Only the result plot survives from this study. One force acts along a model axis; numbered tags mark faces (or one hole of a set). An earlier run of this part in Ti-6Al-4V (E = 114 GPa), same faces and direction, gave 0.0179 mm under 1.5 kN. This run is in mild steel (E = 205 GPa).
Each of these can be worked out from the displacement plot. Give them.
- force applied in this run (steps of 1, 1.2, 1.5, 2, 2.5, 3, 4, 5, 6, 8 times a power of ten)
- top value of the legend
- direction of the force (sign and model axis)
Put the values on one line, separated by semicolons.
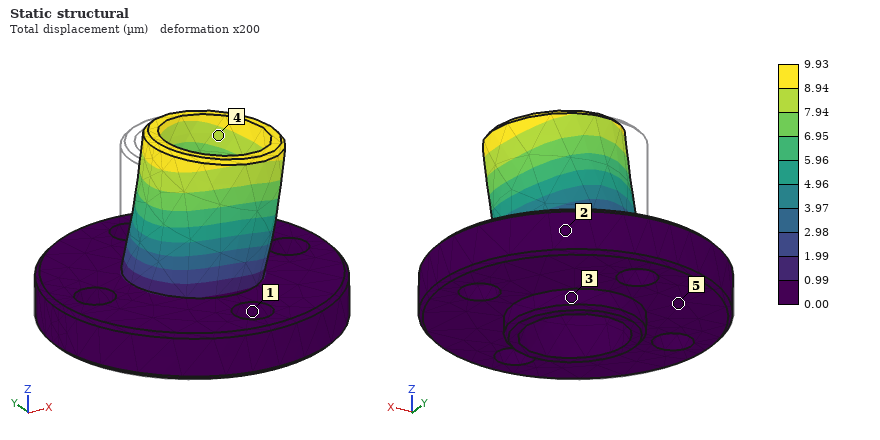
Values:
1.5 kN; 9.93 µm; +X
